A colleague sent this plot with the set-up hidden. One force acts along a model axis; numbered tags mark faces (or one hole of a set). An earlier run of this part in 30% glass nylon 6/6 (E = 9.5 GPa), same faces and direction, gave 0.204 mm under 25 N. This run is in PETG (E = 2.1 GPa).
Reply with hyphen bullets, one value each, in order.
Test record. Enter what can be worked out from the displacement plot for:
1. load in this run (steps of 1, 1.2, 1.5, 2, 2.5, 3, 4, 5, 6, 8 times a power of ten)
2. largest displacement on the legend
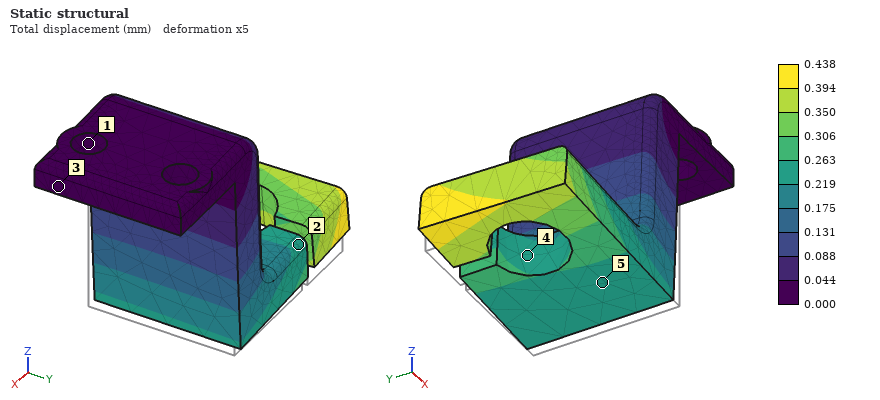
- 12 N
- 0.438 mm
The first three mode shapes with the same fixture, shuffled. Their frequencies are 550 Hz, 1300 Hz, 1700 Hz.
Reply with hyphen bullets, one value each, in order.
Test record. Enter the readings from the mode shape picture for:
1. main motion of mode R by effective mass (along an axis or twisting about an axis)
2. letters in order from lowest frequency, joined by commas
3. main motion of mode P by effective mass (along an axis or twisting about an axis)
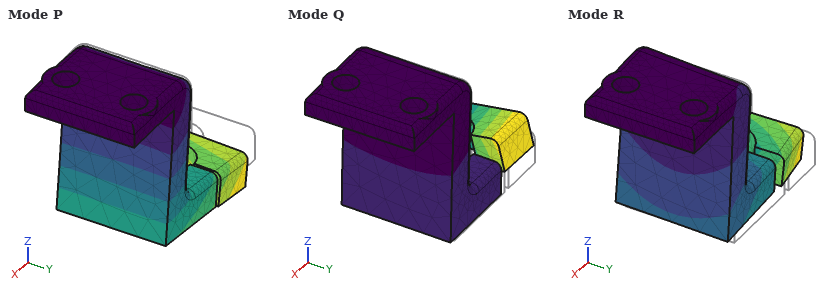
- along Y
- P, R, Q
- along X
